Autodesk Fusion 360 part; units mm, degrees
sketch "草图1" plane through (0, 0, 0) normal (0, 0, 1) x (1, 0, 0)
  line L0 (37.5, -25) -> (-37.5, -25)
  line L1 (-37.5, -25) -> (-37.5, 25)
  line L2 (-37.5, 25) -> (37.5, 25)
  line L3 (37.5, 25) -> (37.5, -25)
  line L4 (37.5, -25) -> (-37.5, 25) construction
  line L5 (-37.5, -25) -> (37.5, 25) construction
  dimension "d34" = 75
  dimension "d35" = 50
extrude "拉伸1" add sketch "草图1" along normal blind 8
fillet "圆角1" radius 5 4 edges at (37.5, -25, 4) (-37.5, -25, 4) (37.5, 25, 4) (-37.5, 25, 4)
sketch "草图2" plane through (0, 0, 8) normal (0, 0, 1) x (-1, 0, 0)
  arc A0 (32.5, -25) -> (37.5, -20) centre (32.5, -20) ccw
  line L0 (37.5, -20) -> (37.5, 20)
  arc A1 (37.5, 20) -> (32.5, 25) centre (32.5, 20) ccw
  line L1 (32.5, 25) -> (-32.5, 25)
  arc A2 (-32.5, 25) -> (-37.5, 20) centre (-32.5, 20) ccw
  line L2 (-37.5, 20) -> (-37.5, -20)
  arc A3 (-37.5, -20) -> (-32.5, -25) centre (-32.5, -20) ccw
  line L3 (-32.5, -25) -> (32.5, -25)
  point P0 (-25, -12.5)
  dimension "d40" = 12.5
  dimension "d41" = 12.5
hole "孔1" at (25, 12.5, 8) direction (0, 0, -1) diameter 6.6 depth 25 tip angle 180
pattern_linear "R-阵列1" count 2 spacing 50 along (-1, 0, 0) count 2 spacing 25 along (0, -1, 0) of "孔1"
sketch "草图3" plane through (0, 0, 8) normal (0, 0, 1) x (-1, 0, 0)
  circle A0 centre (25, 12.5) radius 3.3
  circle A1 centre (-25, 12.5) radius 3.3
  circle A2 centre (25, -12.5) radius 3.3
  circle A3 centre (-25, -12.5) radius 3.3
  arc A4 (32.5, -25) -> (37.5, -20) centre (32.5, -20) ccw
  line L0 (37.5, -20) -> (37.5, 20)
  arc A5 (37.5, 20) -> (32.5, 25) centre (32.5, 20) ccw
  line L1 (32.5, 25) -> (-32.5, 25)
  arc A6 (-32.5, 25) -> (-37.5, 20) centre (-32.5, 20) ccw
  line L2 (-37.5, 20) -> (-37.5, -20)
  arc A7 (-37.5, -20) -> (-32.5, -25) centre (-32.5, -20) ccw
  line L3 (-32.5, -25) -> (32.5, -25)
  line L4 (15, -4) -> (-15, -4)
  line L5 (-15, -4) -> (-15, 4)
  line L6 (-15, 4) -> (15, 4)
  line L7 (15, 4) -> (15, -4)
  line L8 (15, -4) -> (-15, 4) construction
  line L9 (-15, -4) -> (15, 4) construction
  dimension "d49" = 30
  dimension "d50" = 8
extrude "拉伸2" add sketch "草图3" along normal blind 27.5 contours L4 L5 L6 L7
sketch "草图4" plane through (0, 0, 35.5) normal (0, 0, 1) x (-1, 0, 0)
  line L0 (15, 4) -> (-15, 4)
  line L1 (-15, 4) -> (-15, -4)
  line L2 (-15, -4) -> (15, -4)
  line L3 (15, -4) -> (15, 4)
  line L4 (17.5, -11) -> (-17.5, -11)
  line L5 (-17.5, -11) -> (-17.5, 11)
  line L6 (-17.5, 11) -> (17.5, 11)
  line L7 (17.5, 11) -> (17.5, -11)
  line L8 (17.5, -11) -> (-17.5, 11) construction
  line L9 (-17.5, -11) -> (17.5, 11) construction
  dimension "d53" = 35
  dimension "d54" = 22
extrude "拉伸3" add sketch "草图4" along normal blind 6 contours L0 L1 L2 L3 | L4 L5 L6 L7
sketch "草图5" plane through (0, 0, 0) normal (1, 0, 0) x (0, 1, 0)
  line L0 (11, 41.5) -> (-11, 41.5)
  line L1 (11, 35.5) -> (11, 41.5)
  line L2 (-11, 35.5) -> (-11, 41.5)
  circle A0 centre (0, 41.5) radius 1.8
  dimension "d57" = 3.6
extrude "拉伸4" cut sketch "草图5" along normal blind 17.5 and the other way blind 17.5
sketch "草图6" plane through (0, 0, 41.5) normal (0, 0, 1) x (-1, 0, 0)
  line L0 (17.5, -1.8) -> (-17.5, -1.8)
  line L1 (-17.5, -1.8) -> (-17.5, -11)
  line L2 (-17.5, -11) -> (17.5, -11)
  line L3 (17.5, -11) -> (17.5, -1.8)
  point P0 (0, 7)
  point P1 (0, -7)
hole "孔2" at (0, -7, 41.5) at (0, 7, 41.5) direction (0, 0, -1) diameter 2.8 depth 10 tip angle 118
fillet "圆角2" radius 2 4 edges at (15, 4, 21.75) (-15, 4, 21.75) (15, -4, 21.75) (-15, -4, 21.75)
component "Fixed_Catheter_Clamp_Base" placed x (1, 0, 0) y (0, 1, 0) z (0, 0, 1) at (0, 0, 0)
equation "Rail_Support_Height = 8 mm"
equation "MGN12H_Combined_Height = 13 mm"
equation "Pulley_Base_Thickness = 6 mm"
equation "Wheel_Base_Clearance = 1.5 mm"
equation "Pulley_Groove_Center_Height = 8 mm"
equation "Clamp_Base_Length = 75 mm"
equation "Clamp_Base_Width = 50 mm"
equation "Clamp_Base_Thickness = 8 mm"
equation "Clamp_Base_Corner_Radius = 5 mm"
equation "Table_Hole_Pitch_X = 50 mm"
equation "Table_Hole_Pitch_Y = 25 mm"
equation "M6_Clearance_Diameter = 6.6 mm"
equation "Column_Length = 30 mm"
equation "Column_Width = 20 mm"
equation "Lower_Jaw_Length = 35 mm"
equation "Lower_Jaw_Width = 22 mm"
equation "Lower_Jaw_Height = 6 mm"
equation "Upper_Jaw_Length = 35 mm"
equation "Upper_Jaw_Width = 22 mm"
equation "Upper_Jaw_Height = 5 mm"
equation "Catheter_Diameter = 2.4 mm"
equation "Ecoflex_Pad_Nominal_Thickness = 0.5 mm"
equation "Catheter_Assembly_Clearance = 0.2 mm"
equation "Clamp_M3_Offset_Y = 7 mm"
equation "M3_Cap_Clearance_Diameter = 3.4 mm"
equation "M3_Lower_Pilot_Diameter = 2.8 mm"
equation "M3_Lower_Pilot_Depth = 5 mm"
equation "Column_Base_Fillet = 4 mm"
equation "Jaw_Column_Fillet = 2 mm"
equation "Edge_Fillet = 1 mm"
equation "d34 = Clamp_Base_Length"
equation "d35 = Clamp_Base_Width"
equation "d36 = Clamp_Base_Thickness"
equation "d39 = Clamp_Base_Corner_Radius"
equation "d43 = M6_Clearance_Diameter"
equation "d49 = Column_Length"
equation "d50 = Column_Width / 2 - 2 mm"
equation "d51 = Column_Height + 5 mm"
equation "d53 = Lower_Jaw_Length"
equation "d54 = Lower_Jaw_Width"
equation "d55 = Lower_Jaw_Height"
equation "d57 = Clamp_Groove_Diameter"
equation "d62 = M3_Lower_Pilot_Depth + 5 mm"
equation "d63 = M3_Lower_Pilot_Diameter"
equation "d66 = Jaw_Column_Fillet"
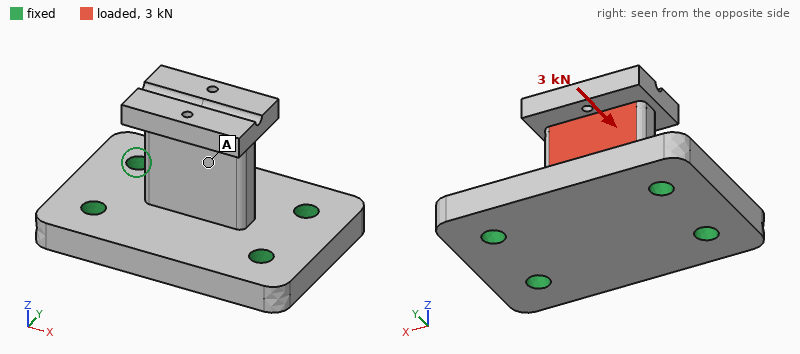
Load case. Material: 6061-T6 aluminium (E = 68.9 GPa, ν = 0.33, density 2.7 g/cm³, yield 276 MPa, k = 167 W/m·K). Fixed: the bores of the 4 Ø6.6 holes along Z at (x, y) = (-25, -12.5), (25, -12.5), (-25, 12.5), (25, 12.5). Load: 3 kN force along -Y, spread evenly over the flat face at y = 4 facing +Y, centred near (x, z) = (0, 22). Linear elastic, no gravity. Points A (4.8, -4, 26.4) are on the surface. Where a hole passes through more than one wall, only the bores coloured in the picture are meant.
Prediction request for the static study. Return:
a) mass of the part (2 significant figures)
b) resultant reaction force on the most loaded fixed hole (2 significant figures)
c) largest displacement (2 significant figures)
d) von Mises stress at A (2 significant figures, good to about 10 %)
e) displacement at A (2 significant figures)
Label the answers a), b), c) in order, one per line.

a) 110 g
b) 1.3 kN
c) 0.22 mm
d) 17 MPa
e) 0.11 mm
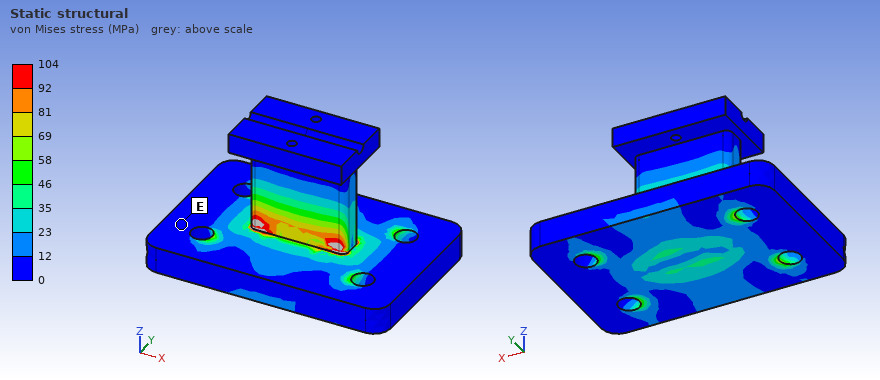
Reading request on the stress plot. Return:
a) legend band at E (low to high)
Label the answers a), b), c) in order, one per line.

a) 0 to 12 MPa
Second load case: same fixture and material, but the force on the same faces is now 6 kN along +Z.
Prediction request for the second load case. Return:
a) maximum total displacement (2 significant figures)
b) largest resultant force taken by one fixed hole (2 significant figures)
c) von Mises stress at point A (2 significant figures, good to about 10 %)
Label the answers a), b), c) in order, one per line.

a) 0.15 mm
b) 2.0 kN
c) 18 MPa
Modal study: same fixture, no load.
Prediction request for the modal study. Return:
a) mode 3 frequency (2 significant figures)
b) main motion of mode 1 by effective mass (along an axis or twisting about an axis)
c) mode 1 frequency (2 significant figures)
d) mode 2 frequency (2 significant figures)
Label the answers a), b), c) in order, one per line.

a) 7400 Hz
b) along Y
c) 3100 Hz
d) 7300 Hz
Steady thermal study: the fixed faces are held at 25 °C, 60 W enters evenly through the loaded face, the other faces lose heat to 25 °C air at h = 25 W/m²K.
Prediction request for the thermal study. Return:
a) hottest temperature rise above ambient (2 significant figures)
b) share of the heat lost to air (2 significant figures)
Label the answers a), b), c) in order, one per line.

a) 33 K
b) 5.2 %
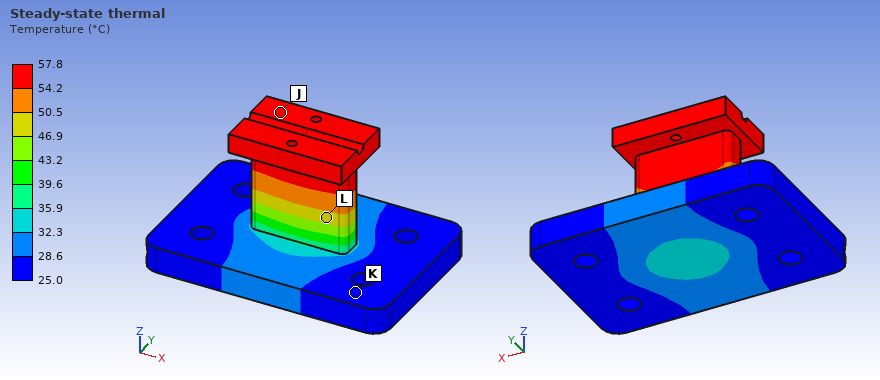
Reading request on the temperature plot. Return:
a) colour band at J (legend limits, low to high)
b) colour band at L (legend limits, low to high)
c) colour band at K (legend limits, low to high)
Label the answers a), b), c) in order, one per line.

a) 54.2 to 57.8 °C
b) 46.9 to 50.5 °C
c) 25.0 to 28.6 °C
